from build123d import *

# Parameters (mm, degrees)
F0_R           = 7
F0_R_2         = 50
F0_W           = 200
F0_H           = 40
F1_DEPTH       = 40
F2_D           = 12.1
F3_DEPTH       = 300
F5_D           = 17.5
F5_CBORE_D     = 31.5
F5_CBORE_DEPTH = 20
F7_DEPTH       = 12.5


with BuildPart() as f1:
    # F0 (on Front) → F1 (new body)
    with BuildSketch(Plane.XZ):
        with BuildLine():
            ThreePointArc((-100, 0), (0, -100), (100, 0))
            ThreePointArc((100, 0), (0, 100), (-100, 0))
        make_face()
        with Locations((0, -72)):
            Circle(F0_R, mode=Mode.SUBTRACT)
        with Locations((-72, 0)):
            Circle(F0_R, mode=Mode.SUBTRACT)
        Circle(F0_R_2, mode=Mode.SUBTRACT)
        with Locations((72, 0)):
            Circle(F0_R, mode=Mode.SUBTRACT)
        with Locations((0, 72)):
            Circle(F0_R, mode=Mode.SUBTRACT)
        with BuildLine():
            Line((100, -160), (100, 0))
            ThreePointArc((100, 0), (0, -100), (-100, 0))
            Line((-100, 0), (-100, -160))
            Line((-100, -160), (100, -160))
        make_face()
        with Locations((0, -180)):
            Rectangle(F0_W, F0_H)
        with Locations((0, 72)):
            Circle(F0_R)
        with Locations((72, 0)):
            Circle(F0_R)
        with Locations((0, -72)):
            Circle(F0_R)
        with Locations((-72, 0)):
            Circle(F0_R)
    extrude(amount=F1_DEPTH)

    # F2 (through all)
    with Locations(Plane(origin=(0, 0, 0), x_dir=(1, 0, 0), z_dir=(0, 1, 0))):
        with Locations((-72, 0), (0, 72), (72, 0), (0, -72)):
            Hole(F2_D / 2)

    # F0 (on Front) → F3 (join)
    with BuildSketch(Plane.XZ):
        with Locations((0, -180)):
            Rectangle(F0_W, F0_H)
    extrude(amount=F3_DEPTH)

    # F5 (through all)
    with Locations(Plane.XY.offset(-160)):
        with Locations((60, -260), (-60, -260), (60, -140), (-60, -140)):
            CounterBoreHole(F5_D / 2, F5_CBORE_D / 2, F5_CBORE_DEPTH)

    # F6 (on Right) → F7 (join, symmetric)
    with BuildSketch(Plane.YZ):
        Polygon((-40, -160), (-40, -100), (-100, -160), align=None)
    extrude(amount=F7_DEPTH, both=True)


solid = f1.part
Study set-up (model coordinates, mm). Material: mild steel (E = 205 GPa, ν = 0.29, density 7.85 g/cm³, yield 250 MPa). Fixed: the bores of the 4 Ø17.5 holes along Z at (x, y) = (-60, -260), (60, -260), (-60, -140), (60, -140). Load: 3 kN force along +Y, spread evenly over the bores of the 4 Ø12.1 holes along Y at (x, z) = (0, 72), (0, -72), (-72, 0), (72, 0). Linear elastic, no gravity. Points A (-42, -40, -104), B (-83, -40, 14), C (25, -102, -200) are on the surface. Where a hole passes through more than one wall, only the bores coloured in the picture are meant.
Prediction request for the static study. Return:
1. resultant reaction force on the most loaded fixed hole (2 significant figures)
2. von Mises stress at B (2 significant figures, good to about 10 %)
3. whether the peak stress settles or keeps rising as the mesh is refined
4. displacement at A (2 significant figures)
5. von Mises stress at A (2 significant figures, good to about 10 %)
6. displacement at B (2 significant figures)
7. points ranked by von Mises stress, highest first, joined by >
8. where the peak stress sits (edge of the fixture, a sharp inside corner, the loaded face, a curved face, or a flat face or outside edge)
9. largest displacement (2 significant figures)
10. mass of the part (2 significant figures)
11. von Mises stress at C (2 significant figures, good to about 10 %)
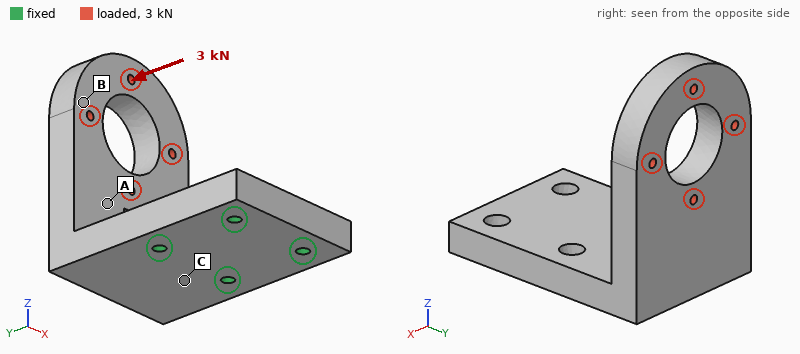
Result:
3.6 kN
1.9 MPa
keeps rising
0.030 mm
4.7 MPa
0.077 mm
C > A > B
edge of the fixture
0.12 mm
31 kg
8.7 MPa
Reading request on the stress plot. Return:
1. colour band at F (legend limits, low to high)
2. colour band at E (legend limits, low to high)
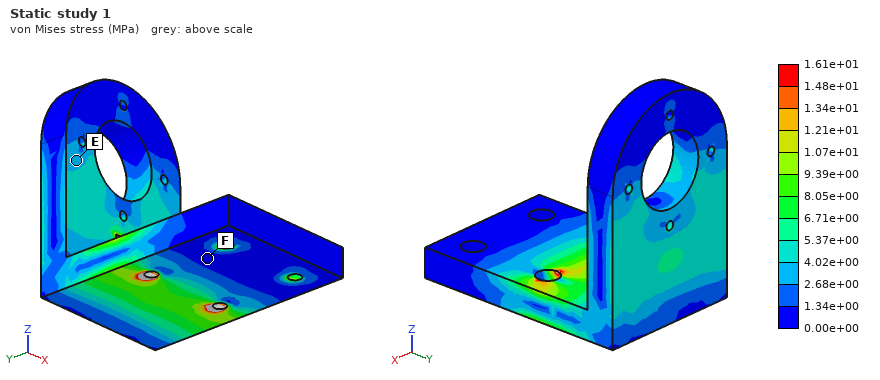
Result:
0.00e+00 to 1.34e+00 MPa
2.68e+00 to 4.02e+00 MPa
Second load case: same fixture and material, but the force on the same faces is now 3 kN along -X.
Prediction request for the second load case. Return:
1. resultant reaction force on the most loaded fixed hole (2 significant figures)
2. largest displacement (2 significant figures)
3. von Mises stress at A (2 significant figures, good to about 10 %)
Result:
5.8 kN
39 µm
1.6 MPa
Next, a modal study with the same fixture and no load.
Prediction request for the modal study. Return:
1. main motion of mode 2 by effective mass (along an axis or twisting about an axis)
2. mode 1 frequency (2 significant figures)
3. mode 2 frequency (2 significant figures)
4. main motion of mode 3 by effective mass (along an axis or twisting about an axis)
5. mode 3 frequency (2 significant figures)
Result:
along X
310 Hz
540 Hz
along Z
960 Hz
